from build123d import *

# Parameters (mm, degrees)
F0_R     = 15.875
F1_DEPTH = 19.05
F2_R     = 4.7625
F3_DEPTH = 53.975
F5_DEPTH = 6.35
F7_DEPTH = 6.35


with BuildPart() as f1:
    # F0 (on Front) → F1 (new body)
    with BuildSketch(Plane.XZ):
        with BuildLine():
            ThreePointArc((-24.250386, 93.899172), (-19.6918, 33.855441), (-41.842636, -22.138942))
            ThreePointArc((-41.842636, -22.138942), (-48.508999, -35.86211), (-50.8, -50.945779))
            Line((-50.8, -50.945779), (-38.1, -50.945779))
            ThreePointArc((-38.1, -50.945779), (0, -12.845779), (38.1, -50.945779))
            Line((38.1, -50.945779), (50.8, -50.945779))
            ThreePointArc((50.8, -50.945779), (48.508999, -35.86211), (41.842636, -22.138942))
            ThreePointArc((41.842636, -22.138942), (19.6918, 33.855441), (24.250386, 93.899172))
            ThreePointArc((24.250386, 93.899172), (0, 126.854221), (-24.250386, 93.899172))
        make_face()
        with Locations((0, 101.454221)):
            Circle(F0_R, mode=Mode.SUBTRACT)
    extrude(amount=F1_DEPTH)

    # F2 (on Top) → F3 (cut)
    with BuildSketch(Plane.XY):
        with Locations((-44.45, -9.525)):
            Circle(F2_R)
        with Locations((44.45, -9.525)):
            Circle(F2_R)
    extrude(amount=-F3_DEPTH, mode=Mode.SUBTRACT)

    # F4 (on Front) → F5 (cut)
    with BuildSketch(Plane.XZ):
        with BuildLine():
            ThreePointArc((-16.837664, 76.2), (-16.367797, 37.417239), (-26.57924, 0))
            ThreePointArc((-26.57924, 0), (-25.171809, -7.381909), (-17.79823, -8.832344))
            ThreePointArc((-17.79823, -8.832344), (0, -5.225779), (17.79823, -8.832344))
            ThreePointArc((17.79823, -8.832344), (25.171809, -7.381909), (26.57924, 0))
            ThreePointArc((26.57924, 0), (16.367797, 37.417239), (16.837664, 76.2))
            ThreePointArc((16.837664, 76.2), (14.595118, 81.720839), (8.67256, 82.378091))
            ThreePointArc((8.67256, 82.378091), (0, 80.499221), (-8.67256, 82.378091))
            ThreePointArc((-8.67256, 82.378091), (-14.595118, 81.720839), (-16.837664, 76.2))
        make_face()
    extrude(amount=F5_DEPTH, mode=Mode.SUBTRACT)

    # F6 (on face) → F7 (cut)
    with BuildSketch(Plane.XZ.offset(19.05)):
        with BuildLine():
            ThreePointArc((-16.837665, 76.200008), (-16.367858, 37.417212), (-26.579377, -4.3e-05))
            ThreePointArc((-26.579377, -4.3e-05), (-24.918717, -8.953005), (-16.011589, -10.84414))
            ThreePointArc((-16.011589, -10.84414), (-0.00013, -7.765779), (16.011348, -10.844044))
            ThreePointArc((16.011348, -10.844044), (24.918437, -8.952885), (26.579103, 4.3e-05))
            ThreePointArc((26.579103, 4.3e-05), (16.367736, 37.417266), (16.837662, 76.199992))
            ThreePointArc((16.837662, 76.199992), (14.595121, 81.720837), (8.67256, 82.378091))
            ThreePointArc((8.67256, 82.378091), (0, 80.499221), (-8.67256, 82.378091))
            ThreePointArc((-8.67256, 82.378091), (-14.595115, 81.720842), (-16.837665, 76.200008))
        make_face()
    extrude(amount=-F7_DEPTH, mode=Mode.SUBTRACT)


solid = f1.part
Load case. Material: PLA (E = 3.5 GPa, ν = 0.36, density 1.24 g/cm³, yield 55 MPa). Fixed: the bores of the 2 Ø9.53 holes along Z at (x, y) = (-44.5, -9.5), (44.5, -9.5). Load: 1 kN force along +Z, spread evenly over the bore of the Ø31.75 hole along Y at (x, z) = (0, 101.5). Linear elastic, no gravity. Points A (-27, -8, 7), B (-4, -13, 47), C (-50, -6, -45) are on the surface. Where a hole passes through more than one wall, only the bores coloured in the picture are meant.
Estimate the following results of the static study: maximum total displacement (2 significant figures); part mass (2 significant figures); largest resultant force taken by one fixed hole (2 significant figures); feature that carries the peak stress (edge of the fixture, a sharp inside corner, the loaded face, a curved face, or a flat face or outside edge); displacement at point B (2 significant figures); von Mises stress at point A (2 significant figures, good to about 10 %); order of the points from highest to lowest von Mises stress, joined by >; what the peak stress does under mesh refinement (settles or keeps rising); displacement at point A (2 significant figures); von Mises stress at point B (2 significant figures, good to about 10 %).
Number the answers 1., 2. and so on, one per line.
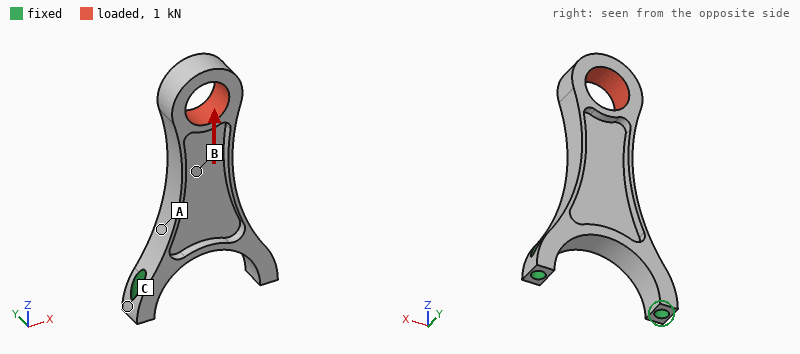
1. 0.16 mm
2. 99 g
3. 610 N
4. edge of the fixture
5. 0.075 mm
6. 3.9 MPa
7. A > B > C
8. keeps rising
9. 0.034 mm
10. 2.9 MPa
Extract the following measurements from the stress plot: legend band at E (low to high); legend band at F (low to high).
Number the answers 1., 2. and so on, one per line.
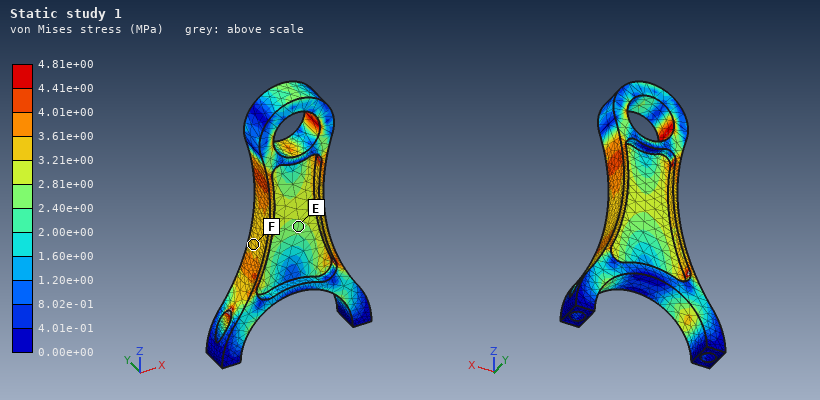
1. 2.40e+00 to 2.81e+00 MPa
2. 3.21e+00 to 3.61e+00 MPa
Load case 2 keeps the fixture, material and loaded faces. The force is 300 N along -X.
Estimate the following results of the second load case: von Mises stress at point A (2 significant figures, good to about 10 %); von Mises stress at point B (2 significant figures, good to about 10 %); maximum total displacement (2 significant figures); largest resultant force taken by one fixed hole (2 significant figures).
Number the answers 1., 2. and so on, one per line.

1. 7.3 MPa
2. 2.7 MPa
3. 0.92 mm
4. 560 N
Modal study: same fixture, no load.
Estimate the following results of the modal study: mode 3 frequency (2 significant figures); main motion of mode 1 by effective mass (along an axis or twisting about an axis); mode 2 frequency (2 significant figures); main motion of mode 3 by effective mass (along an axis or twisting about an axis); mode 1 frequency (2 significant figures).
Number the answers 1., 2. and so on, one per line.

1. 570 Hz
2. along Y
3. 440 Hz
4. along X
5. 130 Hz
